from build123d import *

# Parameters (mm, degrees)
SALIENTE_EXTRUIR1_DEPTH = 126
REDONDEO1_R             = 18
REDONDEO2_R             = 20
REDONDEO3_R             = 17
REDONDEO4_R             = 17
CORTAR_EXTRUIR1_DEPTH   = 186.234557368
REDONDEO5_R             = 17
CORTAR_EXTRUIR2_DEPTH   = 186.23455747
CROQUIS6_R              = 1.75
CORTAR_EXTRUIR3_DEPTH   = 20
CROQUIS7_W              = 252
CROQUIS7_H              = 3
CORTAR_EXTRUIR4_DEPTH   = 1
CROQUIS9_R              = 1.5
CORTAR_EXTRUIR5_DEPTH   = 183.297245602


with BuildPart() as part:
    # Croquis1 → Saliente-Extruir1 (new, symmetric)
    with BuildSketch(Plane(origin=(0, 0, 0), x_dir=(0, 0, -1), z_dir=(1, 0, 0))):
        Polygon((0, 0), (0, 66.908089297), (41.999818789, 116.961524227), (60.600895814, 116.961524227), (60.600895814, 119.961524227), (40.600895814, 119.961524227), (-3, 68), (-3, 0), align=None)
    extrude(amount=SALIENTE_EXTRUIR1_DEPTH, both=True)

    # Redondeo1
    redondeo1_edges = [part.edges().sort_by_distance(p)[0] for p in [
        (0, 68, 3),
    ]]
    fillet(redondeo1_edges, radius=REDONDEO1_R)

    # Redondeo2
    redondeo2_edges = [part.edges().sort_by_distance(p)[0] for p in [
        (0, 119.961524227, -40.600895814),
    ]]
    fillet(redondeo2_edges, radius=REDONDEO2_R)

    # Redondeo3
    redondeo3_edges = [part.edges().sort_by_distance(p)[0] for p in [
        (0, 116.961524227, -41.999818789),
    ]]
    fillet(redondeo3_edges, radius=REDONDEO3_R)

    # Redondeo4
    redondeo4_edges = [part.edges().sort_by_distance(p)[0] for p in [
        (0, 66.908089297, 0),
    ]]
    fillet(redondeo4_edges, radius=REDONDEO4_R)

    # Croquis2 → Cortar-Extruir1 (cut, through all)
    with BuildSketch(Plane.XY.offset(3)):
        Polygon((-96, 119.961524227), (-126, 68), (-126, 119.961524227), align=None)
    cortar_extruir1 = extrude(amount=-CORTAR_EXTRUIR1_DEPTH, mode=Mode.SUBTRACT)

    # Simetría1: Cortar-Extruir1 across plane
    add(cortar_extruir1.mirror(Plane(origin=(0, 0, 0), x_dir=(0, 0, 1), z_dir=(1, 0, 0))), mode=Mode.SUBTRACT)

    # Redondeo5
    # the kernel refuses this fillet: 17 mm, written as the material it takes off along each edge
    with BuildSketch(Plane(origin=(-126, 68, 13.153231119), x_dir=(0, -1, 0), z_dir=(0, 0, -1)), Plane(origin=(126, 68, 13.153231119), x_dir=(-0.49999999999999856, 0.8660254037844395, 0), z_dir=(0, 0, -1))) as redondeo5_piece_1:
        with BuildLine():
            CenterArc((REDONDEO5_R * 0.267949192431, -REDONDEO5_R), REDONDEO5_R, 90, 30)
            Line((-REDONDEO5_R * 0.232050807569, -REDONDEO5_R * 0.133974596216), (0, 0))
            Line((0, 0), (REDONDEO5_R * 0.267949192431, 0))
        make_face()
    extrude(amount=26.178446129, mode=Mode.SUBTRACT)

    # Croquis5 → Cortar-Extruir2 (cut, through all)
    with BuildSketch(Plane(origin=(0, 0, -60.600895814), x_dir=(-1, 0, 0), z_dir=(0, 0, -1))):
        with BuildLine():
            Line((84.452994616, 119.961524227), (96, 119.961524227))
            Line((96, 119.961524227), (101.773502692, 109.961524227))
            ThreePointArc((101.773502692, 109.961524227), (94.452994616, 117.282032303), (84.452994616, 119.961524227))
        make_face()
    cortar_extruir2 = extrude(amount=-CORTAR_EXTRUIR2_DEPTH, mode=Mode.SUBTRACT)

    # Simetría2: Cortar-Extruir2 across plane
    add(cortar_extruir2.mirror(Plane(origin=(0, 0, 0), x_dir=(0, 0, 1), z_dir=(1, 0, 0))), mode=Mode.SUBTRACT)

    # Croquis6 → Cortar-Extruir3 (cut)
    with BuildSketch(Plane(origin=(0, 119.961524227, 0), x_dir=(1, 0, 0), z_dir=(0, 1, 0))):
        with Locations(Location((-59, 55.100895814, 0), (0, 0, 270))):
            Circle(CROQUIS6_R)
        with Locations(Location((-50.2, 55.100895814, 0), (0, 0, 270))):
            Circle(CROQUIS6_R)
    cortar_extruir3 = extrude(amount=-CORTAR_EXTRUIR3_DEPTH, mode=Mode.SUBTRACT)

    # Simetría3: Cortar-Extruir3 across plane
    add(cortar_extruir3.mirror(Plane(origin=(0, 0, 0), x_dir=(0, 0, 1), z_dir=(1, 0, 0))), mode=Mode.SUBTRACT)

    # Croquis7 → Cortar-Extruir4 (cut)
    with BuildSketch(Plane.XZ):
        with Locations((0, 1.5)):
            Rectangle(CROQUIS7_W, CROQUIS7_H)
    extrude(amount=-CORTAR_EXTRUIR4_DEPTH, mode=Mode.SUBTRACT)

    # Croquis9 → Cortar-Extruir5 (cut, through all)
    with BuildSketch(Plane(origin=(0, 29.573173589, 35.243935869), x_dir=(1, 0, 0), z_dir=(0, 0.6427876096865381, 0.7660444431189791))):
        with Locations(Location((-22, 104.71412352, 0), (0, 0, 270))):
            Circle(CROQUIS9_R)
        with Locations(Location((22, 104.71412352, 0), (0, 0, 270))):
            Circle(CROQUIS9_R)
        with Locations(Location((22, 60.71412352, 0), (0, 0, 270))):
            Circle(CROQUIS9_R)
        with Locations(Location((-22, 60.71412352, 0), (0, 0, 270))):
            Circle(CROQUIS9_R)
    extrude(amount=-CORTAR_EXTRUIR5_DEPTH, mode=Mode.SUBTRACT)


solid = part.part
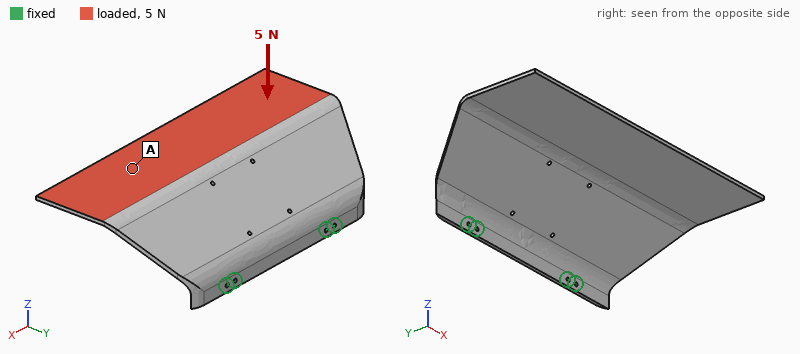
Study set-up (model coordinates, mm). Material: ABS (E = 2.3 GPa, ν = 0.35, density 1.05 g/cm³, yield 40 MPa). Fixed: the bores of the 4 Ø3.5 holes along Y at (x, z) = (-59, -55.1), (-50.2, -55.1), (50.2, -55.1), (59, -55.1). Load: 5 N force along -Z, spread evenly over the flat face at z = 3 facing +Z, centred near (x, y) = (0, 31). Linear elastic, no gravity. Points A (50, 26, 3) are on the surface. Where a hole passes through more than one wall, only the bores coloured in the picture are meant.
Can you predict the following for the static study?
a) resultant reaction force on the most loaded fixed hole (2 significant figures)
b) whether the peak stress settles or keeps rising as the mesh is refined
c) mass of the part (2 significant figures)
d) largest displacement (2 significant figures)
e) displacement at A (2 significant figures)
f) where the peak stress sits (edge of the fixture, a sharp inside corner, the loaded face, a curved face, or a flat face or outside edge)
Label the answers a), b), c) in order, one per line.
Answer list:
a) 3.5 N
b) keeps rising
c) 110 g
d) 3.4 mm
e) 2.6 mm
f) edge of the fixture
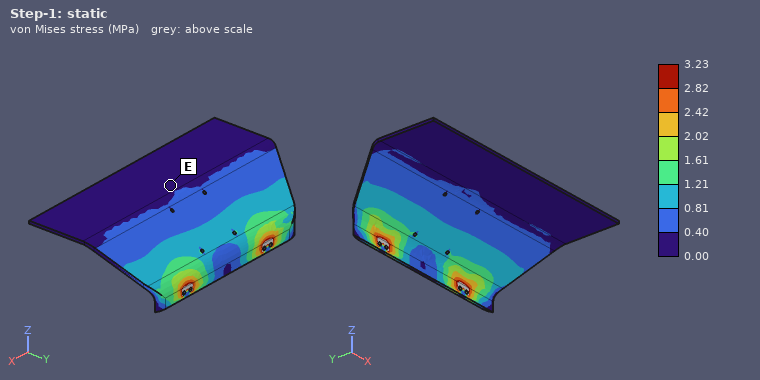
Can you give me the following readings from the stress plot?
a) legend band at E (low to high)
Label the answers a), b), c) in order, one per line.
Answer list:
a) 0.00 to 0.40 MPa
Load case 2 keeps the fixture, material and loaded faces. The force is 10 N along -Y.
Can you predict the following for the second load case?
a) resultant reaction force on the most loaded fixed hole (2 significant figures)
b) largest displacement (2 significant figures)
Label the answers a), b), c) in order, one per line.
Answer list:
a) 3.3 N
b) 3.2 mm
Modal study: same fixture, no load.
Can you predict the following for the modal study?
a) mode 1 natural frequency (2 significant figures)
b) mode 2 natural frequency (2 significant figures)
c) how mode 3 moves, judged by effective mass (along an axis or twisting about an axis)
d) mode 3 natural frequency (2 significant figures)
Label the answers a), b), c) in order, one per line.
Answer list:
a) 28 Hz
b) 47 Hz
c) along Y
d) 160 Hz
